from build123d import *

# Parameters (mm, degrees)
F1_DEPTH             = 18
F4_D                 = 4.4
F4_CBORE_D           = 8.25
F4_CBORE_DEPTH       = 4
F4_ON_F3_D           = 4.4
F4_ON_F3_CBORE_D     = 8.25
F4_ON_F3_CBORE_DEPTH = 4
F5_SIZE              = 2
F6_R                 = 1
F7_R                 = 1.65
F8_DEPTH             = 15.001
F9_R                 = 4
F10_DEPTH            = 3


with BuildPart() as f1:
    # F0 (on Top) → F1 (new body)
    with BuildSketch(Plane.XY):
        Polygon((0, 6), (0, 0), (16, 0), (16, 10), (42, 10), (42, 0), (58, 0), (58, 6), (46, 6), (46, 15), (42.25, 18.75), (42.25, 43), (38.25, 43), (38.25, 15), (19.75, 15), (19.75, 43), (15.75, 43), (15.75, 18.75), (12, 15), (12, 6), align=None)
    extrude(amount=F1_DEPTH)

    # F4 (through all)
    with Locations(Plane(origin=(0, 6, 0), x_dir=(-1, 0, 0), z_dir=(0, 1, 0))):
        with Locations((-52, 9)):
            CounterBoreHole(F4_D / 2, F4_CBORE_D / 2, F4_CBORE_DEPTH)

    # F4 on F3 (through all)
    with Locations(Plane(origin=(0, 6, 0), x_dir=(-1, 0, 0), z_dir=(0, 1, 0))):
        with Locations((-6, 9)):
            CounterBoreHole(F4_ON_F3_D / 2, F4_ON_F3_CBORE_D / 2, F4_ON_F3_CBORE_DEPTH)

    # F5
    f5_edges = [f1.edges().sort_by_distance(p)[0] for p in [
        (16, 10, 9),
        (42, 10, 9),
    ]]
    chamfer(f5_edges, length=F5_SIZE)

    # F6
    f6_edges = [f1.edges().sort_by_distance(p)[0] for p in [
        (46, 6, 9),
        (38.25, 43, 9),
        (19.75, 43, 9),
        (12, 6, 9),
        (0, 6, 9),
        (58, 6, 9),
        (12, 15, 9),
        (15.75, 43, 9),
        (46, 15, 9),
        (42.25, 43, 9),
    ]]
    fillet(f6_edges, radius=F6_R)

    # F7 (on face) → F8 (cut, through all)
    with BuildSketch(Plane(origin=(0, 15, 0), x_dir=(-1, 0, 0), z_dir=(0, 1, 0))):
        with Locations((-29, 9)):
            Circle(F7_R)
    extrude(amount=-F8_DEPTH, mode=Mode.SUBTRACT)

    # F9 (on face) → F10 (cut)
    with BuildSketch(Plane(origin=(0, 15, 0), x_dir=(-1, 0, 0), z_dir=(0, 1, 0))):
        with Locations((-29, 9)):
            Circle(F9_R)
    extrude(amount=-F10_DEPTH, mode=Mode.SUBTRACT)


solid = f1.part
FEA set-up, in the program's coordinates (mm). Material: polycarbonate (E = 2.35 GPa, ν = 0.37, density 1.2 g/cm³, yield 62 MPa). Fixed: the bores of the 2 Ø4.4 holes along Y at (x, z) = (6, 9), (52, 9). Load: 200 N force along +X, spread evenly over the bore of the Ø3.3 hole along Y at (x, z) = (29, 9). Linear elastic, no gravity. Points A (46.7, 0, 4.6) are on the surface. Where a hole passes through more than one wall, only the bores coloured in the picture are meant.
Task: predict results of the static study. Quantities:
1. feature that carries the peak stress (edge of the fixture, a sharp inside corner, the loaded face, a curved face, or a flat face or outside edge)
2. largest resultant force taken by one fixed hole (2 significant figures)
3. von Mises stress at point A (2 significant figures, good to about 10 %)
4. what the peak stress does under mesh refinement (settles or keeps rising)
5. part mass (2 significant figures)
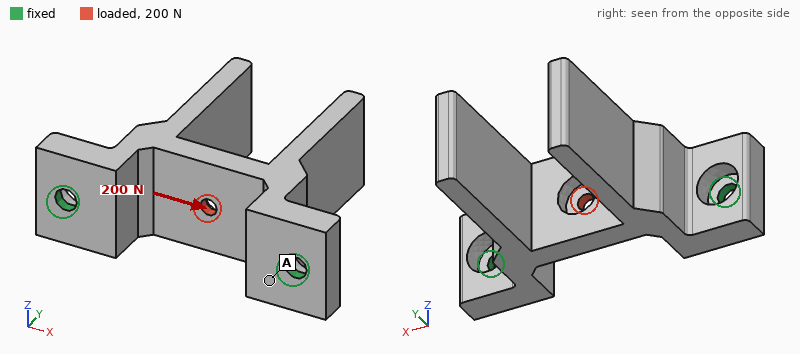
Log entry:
a sharp inside corner
110 N
1.8 MPa
keeps rising
13 g
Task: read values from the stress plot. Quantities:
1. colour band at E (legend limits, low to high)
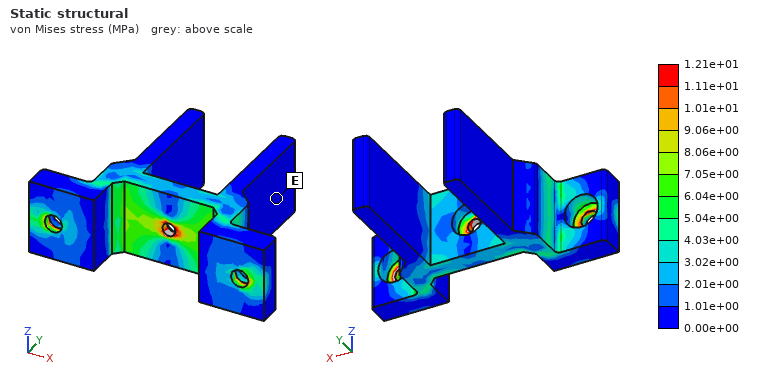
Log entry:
0.00e+00 to 1.01e+00 MPa
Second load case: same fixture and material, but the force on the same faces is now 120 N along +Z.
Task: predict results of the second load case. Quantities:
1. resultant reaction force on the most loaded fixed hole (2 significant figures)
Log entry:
60 N
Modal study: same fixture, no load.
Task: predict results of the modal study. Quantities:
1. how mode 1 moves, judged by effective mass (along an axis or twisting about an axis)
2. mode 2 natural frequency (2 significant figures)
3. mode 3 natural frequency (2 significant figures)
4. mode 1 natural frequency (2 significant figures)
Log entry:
along Z
1100 Hz
1100 Hz
590 Hz
